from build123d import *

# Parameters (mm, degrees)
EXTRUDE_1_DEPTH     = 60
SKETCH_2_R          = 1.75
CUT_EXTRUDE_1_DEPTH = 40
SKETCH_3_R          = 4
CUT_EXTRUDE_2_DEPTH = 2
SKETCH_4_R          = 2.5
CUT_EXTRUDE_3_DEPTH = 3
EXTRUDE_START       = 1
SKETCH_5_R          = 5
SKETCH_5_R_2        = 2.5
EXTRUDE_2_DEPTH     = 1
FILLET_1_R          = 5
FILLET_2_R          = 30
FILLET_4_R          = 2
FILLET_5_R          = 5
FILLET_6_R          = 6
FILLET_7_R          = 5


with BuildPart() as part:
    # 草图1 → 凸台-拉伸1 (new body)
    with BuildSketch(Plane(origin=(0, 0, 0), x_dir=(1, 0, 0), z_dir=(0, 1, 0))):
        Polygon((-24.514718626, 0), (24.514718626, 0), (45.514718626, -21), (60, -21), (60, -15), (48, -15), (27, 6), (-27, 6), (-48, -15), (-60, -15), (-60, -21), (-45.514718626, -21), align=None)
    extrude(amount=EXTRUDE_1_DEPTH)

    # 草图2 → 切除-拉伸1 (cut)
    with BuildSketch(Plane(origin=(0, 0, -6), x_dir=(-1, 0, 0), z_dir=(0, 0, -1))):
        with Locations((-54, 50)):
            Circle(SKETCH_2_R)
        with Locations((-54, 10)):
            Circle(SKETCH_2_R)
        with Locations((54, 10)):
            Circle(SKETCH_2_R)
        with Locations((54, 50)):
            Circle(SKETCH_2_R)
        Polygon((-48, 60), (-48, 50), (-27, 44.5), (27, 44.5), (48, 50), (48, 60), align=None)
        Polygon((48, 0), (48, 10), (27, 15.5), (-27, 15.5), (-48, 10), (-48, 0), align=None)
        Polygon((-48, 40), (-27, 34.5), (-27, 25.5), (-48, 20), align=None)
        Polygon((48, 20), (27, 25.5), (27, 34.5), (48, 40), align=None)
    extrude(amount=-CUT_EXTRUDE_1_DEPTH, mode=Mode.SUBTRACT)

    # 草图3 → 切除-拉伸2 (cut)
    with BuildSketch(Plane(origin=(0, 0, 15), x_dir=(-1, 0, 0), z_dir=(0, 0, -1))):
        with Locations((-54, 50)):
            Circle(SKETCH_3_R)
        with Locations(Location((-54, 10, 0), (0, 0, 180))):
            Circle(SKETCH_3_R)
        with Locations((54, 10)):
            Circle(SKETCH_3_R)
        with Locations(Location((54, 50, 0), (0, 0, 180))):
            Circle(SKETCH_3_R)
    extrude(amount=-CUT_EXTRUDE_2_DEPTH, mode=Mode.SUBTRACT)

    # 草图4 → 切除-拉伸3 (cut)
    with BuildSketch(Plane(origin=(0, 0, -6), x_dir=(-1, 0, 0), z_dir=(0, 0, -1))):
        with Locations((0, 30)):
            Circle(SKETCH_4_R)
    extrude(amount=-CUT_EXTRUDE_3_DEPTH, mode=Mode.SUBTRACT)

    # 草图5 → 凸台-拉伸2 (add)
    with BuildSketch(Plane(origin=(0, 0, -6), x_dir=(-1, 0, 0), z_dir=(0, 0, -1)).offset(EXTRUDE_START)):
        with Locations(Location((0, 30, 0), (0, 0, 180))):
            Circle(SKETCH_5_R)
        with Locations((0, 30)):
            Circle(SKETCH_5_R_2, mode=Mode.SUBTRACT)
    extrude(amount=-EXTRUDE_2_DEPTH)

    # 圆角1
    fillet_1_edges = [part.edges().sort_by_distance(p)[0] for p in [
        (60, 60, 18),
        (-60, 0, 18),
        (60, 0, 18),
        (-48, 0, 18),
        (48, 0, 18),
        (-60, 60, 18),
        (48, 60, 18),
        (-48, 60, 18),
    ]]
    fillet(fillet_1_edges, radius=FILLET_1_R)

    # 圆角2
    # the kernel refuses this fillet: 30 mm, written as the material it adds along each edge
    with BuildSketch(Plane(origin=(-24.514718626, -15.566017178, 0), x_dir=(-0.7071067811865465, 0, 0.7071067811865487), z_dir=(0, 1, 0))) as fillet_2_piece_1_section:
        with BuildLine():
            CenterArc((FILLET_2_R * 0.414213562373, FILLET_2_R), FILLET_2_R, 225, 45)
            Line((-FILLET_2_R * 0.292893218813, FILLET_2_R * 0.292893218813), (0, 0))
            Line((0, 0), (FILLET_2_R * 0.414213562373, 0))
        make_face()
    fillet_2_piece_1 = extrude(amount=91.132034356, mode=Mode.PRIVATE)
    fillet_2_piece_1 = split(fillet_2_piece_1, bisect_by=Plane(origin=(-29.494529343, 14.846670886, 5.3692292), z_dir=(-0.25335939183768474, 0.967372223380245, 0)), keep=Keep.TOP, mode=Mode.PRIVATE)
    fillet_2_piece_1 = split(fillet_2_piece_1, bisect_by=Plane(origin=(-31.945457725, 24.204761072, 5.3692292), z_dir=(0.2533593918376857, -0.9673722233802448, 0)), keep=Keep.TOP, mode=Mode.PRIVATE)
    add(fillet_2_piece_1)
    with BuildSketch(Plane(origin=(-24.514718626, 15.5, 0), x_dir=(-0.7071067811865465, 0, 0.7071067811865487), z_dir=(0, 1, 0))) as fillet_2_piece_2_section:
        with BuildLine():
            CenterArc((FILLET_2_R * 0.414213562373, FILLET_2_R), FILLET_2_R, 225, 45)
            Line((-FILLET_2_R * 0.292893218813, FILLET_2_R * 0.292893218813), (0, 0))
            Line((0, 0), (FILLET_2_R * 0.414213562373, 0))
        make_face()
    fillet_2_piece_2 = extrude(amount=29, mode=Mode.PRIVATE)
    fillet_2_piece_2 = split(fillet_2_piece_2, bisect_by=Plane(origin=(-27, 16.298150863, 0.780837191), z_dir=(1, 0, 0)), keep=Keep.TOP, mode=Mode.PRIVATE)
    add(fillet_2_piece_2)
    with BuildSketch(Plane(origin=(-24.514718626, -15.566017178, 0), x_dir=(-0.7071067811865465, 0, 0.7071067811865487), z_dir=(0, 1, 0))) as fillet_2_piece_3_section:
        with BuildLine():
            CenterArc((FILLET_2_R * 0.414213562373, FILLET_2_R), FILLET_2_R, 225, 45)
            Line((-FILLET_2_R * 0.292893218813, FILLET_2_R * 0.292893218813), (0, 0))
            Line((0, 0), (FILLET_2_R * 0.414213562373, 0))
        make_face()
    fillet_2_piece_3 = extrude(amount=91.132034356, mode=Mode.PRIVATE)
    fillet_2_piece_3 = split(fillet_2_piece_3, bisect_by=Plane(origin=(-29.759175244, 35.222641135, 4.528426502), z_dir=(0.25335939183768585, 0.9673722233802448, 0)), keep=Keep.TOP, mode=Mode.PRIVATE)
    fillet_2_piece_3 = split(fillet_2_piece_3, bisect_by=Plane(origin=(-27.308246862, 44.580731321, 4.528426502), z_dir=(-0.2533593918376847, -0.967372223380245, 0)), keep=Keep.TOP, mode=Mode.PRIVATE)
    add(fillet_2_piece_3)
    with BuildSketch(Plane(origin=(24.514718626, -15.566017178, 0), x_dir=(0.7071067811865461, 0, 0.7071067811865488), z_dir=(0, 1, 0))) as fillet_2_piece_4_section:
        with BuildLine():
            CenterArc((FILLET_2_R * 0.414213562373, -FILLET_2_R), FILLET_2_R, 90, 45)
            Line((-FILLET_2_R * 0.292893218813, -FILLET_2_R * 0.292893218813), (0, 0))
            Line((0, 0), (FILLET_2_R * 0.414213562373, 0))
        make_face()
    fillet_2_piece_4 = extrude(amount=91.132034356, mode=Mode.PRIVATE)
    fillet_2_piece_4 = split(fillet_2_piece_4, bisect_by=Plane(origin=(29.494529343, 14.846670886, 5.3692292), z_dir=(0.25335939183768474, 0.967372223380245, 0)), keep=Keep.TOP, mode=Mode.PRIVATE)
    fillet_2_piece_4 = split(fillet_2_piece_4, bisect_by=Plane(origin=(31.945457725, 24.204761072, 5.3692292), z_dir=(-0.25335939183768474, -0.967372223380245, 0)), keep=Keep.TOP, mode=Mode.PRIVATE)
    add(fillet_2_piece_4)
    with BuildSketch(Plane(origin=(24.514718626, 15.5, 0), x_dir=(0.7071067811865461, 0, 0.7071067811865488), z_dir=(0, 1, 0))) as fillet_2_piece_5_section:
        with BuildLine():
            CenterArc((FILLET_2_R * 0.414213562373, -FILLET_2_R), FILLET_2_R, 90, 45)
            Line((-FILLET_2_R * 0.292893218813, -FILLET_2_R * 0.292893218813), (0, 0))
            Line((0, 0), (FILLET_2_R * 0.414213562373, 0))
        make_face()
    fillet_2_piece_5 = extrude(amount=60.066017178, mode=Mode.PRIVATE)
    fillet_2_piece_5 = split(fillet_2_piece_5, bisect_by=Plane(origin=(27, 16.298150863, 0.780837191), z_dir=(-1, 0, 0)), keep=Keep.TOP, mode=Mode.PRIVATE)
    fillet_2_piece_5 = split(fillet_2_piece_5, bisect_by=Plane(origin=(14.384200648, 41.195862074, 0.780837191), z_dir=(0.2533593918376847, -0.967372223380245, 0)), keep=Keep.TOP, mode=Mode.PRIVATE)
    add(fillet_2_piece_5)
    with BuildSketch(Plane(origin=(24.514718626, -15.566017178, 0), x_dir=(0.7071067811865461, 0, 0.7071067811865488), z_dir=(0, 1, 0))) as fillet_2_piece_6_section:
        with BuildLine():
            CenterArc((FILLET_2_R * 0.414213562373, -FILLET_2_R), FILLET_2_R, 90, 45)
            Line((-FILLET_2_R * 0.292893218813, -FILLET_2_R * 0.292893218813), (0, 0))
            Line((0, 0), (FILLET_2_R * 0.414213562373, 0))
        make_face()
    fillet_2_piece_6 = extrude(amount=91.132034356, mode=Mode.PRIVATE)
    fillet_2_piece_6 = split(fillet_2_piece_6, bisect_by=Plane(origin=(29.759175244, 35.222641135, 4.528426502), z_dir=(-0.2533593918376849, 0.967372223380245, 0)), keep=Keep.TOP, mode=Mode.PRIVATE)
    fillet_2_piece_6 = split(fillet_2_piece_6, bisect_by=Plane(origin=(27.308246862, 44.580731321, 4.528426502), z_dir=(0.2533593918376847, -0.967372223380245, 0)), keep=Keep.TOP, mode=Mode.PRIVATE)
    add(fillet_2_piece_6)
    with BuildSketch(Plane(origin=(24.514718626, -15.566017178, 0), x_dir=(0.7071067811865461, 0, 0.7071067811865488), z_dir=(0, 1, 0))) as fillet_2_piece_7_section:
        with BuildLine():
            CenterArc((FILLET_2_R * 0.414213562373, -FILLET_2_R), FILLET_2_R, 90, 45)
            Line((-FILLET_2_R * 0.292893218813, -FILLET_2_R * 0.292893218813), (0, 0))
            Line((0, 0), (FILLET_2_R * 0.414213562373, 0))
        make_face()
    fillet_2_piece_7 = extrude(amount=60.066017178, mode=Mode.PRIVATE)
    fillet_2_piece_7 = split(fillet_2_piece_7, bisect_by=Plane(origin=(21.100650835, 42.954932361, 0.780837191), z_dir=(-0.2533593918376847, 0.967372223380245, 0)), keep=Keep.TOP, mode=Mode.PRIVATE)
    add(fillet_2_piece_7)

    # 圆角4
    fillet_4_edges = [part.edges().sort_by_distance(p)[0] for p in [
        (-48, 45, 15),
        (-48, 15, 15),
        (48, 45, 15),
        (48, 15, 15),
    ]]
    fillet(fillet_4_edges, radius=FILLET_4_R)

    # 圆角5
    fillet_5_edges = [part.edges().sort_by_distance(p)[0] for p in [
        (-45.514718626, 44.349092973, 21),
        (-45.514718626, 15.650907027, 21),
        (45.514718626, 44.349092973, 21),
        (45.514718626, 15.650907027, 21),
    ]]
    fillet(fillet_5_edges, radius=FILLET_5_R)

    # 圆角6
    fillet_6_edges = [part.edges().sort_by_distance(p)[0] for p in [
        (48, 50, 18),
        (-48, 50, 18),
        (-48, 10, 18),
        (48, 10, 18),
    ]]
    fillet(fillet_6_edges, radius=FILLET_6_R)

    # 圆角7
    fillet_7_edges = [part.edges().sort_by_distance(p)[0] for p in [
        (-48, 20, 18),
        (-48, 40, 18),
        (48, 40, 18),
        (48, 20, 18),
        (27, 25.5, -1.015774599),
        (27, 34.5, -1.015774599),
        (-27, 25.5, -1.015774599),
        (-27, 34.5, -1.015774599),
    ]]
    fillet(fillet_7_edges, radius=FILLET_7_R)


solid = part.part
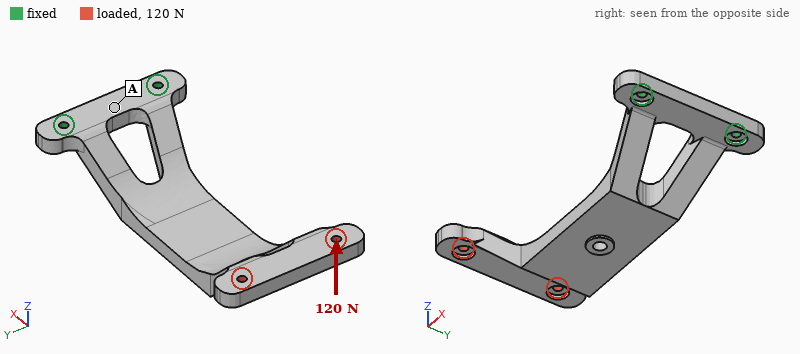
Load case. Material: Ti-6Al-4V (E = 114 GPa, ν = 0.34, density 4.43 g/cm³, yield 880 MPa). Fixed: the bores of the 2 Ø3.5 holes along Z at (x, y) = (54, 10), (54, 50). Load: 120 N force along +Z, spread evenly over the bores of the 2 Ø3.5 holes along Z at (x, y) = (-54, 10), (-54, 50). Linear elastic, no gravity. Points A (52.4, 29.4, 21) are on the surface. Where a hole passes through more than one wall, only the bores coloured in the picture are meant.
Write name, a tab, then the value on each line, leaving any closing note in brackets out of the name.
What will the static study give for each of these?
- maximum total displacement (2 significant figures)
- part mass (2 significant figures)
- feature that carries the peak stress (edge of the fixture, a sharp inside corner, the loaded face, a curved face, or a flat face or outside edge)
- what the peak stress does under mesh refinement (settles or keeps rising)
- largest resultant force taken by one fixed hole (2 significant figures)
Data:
maximum total displacement	1.3 mm
part mass	110 g
feature that carries the peak stress	edge of the fixture
what the peak stress does under mesh refinement	keeps rising
largest resultant force taken by one fixed hole	77 N
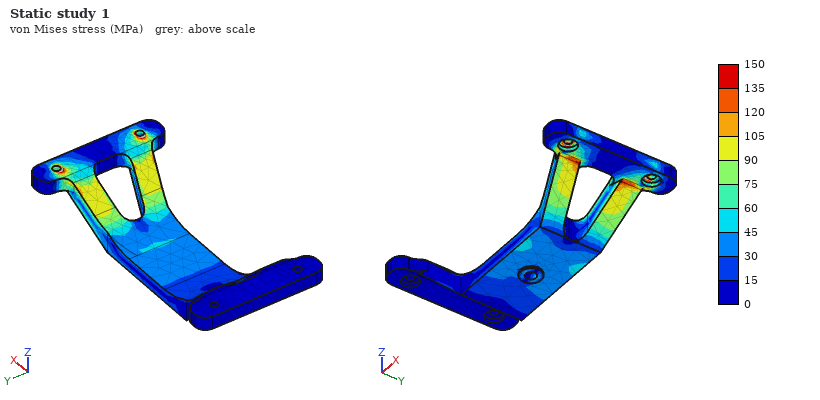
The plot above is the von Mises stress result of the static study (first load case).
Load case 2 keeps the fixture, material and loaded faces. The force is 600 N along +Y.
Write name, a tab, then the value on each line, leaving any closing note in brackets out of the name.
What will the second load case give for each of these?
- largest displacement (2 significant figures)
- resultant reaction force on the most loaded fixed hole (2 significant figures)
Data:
largest displacement	1.5 mm
resultant reaction force on the most loaded fixed hole	1.6 kN
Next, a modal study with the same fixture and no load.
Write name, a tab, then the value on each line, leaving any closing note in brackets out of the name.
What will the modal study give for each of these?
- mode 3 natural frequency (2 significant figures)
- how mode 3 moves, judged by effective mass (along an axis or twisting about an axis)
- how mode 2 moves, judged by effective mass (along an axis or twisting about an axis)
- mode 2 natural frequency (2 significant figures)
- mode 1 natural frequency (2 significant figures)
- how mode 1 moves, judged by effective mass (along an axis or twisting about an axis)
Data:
mode 3 natural frequency	1200 Hz
how mode 3 moves, judged by effective mass	along X
how mode 2 moves, judged by effective mass	along Y
mode 2 natural frequency	610 Hz
mode 1 natural frequency	260 Hz
how mode 1 moves, judged by effective mass	along Z
